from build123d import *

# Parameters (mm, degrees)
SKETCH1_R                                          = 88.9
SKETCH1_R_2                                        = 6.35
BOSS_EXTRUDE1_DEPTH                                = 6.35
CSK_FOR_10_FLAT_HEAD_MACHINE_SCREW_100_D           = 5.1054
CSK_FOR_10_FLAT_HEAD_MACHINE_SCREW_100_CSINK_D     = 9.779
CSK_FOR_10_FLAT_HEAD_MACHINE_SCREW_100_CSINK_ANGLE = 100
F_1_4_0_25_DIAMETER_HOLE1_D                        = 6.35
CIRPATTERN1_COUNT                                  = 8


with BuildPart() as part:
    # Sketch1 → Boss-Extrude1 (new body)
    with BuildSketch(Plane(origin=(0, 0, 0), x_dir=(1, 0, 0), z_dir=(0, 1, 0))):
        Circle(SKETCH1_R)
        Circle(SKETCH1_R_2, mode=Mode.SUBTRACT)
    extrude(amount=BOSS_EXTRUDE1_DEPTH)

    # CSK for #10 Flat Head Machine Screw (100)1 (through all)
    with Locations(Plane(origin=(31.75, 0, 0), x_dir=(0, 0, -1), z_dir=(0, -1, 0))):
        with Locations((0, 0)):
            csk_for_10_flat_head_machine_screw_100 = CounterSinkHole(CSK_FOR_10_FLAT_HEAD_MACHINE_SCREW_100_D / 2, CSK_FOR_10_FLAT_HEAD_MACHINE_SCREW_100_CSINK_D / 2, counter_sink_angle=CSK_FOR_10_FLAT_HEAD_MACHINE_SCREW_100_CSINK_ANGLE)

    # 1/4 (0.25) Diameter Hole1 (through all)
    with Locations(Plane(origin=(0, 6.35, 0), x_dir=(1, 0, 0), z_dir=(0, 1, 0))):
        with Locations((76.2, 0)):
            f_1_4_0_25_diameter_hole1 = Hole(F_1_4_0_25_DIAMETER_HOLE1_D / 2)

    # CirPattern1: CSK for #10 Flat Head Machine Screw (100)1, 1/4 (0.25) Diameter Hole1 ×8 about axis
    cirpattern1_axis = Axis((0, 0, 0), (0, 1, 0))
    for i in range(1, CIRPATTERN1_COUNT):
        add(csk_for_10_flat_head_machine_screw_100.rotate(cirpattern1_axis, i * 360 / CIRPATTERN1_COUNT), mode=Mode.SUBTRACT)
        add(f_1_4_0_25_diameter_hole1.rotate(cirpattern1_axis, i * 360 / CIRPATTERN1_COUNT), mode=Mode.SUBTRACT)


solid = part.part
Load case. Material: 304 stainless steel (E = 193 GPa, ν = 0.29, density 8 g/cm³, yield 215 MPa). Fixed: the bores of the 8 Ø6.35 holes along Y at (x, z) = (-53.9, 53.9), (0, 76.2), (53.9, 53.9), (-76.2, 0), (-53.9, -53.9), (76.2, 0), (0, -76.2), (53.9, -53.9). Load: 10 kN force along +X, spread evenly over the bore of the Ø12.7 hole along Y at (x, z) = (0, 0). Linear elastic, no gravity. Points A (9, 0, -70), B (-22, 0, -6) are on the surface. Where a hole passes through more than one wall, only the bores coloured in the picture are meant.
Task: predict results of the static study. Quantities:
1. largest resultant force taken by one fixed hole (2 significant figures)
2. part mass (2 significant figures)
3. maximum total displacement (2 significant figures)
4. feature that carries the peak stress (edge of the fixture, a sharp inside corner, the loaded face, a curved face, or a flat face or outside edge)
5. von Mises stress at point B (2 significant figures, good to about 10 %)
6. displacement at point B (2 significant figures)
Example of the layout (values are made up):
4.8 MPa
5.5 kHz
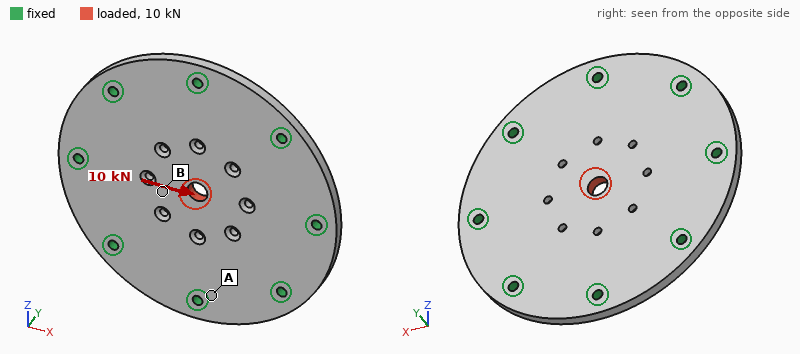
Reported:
2.0 kN
1.2 kg
6.2 µm
the loaded face
21 MPa
3.6 µm
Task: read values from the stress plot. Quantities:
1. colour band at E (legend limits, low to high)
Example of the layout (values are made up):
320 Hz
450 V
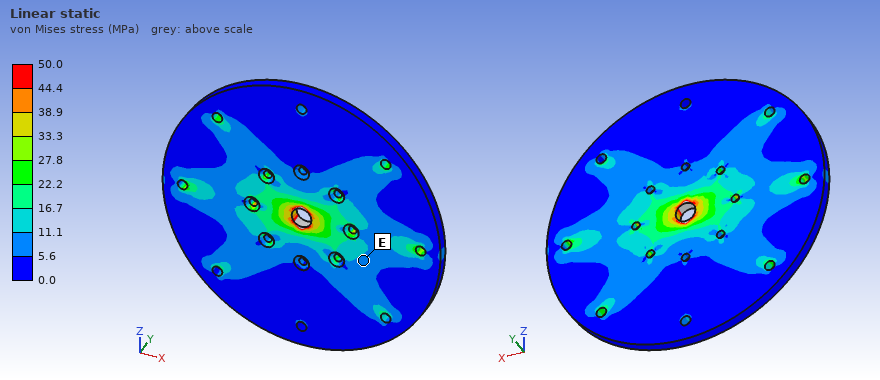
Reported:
5.6 to 11.1 MPa
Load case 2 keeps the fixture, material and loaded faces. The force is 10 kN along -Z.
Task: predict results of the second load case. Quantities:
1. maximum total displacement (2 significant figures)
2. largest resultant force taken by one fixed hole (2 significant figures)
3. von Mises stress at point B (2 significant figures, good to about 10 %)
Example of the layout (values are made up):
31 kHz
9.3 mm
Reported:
6.2 µm
2.0 kN
9.2 MPa
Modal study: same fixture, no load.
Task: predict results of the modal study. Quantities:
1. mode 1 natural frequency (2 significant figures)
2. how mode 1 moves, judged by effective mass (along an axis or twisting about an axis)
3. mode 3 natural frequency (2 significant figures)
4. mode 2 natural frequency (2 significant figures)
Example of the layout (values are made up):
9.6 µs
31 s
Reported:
2300 Hz
along Y
4600 Hz
4600 Hz
